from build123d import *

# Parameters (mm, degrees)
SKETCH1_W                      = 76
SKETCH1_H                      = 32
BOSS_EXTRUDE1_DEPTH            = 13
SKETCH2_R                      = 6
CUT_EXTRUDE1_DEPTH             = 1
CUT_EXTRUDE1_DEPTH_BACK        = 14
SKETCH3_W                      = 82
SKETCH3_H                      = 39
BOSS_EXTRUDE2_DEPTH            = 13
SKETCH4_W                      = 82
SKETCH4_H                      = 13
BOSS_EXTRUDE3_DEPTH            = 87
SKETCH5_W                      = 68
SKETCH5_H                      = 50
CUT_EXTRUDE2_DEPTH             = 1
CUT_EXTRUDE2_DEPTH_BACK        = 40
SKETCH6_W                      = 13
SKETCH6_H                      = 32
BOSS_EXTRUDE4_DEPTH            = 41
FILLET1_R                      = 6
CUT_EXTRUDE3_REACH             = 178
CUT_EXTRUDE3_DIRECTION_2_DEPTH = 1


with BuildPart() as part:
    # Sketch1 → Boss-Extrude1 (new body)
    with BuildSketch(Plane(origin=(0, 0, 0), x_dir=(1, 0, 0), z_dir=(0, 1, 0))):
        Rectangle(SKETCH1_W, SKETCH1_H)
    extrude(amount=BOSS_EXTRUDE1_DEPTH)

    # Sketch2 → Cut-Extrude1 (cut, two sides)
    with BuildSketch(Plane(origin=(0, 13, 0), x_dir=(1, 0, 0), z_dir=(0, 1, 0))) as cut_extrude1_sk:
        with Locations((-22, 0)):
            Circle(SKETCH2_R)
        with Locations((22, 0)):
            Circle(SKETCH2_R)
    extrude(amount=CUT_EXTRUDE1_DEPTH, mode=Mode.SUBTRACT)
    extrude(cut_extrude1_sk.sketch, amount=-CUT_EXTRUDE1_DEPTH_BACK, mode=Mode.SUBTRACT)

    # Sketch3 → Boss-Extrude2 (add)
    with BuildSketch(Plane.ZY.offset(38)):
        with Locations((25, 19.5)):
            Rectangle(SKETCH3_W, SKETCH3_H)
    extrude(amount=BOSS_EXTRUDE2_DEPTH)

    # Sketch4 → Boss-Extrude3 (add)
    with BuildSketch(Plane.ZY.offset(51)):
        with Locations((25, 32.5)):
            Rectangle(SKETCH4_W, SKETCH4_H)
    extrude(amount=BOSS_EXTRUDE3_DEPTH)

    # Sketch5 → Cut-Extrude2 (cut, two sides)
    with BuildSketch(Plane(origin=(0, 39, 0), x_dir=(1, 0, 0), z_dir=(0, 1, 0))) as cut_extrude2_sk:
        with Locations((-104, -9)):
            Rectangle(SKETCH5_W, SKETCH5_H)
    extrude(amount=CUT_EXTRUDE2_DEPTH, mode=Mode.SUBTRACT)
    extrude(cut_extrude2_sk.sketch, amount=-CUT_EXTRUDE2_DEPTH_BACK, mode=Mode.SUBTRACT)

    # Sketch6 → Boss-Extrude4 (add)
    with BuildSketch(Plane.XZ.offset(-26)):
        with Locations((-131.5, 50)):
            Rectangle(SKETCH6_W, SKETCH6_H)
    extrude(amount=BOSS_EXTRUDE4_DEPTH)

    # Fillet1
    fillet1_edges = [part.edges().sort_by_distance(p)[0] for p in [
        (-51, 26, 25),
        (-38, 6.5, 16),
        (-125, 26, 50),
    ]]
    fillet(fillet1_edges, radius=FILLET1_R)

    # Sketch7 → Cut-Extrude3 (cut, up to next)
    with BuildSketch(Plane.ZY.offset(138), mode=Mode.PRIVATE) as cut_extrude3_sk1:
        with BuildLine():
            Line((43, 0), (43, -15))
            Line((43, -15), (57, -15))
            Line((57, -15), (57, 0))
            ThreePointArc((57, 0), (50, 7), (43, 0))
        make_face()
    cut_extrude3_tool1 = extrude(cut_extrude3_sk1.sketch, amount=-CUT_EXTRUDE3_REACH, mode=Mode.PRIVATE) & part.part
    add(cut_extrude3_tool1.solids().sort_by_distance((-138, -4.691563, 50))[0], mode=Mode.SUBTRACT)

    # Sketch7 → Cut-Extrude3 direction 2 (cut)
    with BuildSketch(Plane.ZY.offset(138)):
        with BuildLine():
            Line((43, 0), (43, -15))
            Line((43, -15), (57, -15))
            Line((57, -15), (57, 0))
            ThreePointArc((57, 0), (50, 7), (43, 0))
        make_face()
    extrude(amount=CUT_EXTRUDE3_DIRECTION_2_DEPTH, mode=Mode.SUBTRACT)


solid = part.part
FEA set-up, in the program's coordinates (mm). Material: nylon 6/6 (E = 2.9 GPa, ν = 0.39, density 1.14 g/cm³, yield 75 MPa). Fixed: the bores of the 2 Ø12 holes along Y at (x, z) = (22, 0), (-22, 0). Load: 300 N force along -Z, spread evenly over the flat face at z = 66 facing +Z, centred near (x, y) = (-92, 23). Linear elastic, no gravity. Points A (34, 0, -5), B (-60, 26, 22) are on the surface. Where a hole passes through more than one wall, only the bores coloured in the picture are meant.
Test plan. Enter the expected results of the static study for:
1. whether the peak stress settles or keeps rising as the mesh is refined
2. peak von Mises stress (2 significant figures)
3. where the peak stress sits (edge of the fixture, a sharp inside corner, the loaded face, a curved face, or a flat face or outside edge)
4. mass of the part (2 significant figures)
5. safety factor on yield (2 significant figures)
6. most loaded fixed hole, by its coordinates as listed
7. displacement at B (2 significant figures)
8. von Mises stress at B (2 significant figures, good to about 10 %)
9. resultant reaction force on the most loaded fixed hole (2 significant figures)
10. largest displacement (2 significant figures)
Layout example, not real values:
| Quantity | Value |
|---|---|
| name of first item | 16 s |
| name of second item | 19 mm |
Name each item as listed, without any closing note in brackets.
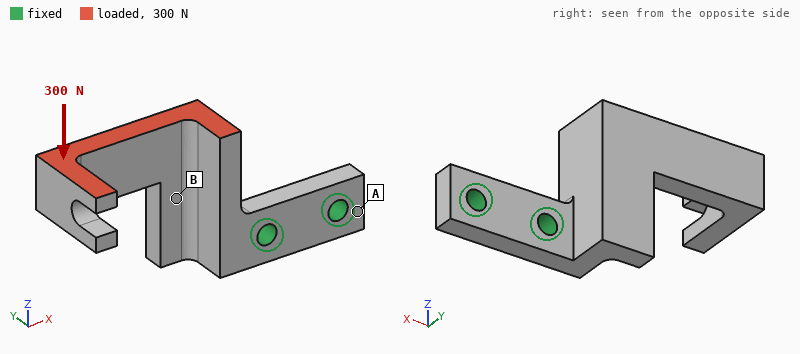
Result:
| Quantity | Value |
|---|---|
| whether the peak stress settles or keeps rising as the mesh is refined | settles |
| peak von Mises stress | 21 MPa |
| where the peak stress sits | a curved face |
| mass of the part | 150 g |
| safety factor on yield | 3.6 |
| most loaded fixed hole, by its coordinates as listed | (-22, 0) |
| displacement at B | 0.38 mm |
| von Mises stress at B | 4.1 MPa |
| resultant reaction force on the most loaded fixed hole | 480 N |
| largest displacement | 2.2 mm |
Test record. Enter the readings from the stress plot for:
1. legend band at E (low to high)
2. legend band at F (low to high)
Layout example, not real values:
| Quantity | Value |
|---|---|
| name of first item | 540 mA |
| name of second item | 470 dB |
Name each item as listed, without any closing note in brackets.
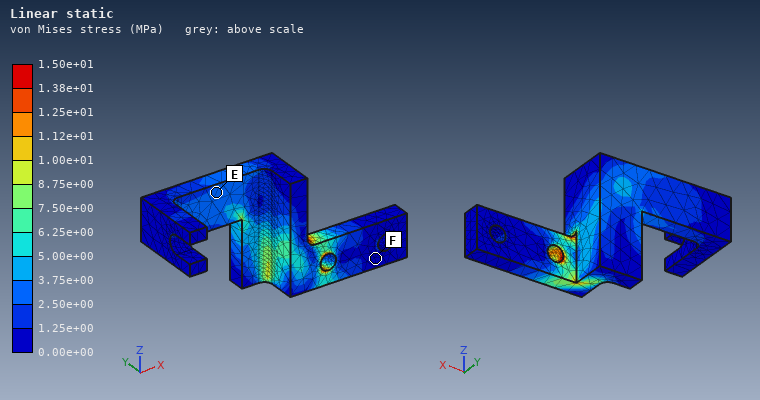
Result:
| Quantity | Value |
|---|---|
| legend band at E | 2.50e+00 to 3.75e+00 MPa |
| legend band at F | 0.00e+00 to 1.25e+00 MPa |
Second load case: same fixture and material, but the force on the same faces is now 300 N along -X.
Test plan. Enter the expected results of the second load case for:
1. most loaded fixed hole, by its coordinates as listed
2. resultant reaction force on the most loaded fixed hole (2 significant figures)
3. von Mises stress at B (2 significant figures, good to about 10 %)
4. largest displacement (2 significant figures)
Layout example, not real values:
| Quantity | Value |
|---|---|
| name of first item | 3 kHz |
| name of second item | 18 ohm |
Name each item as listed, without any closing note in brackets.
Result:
| Quantity | Value |
|---|---|
| most loaded fixed hole, by its coordinates as listed | (-22, 0) |
| resultant reaction force on the most loaded fixed hole | 330 N |
| von Mises stress at B | 2.2 MPa |
| largest displacement | 2.2 mm |
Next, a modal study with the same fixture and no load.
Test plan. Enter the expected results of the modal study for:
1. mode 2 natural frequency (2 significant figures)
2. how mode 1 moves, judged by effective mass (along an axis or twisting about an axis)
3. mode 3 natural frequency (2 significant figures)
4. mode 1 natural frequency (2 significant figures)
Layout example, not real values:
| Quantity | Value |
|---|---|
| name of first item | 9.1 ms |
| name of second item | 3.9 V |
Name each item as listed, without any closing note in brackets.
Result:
| Quantity | Value |
|---|---|
| mode 2 natural frequency | 250 Hz |
| how mode 1 moves, judged by effective mass | along Y |
| mode 3 natural frequency | 470 Hz |
| mode 1 natural frequency | 150 Hz |
